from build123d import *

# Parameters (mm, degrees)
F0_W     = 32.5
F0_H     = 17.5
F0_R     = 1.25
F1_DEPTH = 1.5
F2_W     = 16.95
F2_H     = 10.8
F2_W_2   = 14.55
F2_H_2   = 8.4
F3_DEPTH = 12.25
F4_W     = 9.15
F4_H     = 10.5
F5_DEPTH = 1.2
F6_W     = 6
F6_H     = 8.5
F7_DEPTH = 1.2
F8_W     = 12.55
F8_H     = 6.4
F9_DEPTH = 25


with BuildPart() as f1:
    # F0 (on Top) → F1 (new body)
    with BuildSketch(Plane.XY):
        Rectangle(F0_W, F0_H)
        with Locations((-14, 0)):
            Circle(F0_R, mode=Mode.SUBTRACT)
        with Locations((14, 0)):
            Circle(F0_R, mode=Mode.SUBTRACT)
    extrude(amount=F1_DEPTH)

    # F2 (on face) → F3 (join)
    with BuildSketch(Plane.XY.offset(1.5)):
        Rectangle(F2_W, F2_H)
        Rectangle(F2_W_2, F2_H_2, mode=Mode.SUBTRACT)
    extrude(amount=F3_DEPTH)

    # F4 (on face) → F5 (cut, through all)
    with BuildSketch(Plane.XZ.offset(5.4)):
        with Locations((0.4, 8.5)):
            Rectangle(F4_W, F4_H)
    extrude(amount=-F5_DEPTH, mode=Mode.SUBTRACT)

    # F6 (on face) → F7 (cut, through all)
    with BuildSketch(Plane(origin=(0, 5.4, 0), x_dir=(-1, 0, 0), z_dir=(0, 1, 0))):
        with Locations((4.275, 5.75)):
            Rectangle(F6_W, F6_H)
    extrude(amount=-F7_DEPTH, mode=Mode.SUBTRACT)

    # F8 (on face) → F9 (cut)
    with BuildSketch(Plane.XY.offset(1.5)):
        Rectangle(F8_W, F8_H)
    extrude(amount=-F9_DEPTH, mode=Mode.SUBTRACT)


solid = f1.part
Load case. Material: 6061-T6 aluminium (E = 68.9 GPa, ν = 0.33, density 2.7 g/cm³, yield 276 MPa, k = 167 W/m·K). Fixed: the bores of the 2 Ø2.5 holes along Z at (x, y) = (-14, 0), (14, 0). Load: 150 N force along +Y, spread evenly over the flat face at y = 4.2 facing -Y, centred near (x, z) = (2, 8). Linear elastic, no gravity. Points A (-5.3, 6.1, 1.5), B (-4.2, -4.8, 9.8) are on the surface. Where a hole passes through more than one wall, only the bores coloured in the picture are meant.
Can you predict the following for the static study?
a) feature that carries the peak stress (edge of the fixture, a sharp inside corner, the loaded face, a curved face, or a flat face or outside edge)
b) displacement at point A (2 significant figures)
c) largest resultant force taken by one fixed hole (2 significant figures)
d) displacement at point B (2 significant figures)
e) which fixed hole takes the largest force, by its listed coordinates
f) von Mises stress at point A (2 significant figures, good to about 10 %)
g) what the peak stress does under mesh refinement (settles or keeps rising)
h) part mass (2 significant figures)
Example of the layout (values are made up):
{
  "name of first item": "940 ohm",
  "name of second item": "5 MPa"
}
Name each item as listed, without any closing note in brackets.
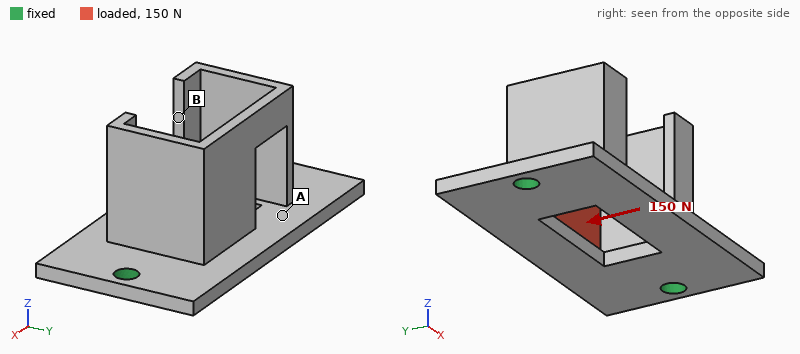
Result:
{
  "feature that carries the peak stress": "edge of the fixture",
  "displacement at point A": "0.043 mm",
  "largest resultant force taken by one fixed hole": "87 N",
  "displacement at point B": "0.059 mm",
  "which fixed hole takes the largest force, by its listed coordinates": "(14, 0)",
  "von Mises stress at point A": "33 MPa",
  "what the peak stress does under mesh refinement": "keeps rising",
  "part mass": "3.5 g"
}
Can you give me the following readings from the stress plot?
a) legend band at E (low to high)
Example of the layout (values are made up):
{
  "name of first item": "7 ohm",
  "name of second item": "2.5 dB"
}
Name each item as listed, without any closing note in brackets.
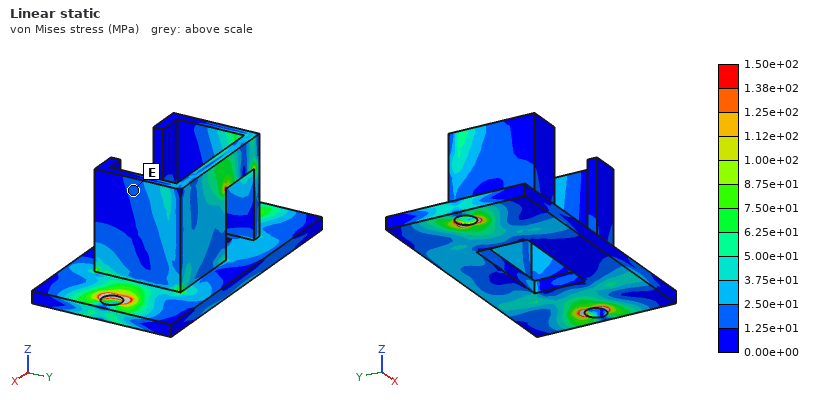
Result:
{
  "legend band at E": "1.25e+01 to 2.50e+01 MPa"
}
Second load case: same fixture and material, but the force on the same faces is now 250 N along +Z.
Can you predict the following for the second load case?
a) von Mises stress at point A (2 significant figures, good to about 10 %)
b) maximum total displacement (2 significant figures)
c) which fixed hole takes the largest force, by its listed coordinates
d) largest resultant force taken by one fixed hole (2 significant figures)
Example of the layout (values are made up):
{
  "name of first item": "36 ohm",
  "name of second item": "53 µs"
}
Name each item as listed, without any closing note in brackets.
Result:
{
  "von Mises stress at point A": "23 MPa",
  "maximum total displacement": "0.11 mm",
  "which fixed hole takes the largest force, by its listed coordinates": "(14, 0)",
  "largest resultant force taken by one fixed hole": "150 N"
}
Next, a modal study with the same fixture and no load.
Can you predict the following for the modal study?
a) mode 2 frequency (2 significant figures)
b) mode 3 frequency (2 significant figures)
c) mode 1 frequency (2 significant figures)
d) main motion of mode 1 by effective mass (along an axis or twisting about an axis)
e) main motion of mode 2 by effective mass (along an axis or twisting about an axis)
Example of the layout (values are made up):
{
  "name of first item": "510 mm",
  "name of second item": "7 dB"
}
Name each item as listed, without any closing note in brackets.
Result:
{
  "mode 2 frequency": "9400 Hz",
  "mode 3 frequency": "11 kHz",
  "mode 1 frequency": "5100 Hz",
  "main motion of mode 1 by effective mass": "along Y",
  "main motion of mode 2 by effective mass": "along Z"
}
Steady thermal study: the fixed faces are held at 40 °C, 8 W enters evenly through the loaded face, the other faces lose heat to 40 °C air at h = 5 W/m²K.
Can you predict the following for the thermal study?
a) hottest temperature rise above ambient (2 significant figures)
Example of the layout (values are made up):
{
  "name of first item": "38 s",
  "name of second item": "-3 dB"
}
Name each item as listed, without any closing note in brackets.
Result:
{
  "hottest temperature rise above ambient": "27 K"
}
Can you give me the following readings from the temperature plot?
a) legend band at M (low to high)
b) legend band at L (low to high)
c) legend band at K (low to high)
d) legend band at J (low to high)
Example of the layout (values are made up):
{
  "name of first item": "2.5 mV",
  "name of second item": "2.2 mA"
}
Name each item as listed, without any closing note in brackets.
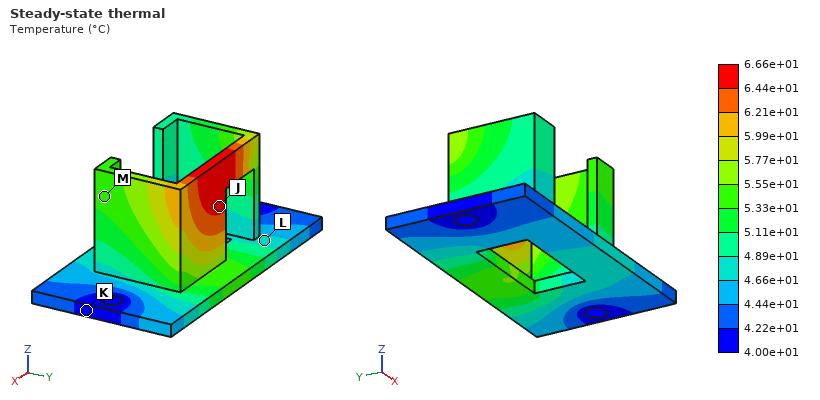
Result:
{
  "legend band at M": "5.33e+01 to 5.55e+01 °C",
  "legend band at L": "4.66e+01 to 4.89e+01 °C",
  "legend band at K": "4.00e+01 to 4.22e+01 °C",
  "legend band at J": "6.44e+01 to 6.66e+01 °C"
}
